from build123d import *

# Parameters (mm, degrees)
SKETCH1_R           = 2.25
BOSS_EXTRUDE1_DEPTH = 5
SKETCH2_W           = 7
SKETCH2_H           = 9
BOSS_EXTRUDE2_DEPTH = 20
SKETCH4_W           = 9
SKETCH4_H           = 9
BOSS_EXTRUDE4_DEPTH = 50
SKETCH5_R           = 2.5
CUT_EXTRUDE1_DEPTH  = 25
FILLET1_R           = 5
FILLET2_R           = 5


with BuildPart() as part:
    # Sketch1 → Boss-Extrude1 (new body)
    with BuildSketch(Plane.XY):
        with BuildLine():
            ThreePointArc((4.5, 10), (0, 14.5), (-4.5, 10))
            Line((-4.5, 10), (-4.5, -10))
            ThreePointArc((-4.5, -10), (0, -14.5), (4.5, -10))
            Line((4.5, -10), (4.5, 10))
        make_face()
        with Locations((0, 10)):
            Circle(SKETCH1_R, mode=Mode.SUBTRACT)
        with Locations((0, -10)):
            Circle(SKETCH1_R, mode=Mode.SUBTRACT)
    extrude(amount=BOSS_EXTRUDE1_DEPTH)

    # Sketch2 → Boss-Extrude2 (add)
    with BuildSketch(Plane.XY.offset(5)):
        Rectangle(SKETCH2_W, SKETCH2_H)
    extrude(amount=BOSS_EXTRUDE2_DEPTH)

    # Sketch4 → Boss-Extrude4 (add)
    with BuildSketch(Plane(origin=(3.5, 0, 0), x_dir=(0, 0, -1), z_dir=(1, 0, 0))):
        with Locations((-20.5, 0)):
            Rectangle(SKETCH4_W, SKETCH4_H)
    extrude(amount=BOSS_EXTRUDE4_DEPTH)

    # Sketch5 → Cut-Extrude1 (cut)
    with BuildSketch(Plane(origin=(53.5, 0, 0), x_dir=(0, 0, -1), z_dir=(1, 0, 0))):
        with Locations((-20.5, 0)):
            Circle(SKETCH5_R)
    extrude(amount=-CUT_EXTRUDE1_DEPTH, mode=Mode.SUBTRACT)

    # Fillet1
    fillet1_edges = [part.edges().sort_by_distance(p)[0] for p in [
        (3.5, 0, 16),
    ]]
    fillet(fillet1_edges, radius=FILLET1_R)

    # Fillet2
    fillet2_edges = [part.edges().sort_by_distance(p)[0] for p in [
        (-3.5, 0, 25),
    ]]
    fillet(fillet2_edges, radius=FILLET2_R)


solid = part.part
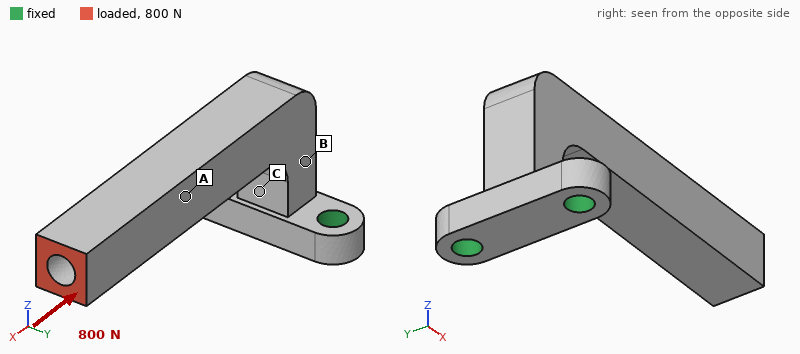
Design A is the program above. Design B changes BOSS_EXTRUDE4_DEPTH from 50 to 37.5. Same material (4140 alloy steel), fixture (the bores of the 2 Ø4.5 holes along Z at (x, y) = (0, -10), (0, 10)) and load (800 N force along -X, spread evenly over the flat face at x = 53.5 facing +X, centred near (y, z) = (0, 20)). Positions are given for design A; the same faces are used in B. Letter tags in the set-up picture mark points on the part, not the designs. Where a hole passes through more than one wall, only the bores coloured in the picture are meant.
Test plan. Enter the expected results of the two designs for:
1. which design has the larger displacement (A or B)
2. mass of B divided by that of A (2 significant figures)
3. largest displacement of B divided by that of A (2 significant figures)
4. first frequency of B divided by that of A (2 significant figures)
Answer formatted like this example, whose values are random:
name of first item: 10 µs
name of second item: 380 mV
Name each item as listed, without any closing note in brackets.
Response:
which design has the larger displacement: A
mass of B divided by that of A: 0.87
largest displacement of B divided by that of A: 0.80
first frequency of B divided by that of A: 1.4
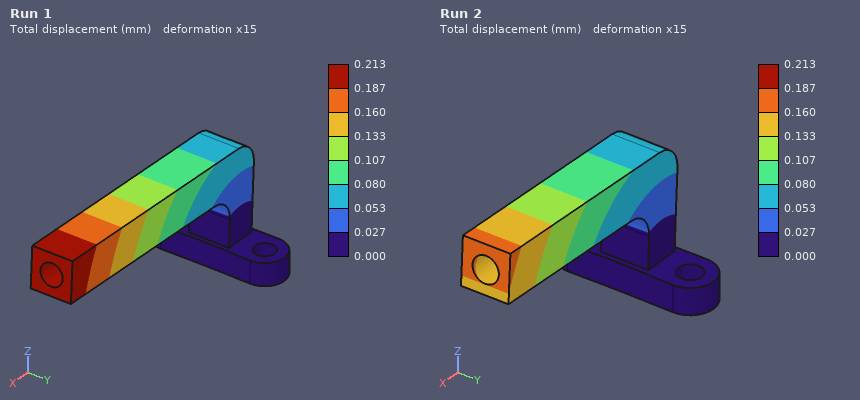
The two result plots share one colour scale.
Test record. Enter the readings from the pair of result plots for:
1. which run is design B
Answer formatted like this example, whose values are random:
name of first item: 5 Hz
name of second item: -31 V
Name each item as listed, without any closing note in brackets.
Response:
which run is design B: Run 2
